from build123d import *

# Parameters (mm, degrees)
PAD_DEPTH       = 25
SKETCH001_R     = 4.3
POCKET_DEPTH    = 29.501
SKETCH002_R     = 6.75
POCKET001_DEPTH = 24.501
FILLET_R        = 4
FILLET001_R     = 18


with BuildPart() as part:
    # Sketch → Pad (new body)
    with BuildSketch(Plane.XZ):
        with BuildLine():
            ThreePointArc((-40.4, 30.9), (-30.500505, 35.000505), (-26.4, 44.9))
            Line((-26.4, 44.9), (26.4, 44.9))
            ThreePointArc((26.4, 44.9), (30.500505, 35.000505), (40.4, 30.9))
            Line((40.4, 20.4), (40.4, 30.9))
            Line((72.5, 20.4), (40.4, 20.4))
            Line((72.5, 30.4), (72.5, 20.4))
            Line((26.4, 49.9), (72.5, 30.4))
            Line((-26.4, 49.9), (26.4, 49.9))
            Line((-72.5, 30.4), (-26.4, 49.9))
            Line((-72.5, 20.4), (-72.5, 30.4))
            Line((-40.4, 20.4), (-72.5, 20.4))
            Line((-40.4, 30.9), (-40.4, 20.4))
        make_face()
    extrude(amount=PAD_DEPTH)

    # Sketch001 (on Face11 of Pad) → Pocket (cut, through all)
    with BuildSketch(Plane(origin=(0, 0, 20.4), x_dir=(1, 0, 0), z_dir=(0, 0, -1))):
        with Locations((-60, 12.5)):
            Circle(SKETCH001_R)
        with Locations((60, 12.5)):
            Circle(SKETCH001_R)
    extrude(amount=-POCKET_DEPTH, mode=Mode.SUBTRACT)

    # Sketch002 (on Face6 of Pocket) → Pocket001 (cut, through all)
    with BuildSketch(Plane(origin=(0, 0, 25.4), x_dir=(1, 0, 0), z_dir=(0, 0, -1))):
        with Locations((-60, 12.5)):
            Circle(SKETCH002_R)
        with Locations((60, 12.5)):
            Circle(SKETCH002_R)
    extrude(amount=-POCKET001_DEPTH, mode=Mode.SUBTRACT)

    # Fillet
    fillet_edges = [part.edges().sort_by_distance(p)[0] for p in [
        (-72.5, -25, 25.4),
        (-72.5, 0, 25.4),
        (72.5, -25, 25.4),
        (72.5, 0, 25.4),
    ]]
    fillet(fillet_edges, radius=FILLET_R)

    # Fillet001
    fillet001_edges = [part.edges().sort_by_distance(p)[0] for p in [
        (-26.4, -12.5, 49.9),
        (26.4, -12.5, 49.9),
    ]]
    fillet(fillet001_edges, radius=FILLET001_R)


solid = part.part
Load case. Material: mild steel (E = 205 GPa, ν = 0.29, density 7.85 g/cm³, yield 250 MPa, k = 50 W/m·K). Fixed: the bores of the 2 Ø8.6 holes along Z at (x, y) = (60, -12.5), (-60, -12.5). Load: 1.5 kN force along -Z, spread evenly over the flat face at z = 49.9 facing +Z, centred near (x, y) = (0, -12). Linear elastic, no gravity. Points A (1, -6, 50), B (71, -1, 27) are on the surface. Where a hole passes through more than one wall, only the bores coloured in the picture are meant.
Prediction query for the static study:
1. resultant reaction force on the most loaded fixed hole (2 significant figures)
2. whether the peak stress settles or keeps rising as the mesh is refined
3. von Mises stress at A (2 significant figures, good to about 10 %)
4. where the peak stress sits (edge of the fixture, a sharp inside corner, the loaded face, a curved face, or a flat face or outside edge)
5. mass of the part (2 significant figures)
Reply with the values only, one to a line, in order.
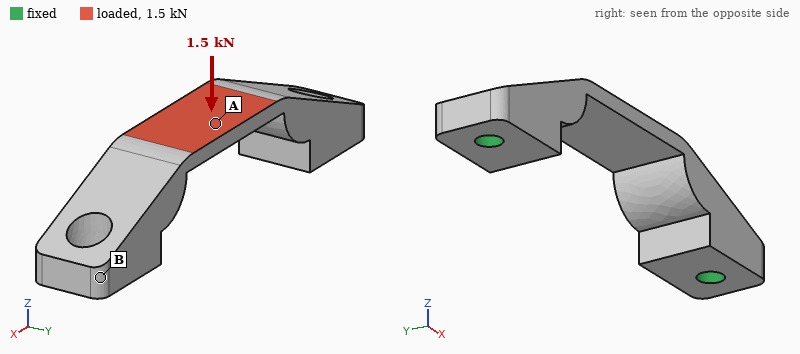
1.4 kN
keeps rising
55 MPa
a sharp inside corner
310 g
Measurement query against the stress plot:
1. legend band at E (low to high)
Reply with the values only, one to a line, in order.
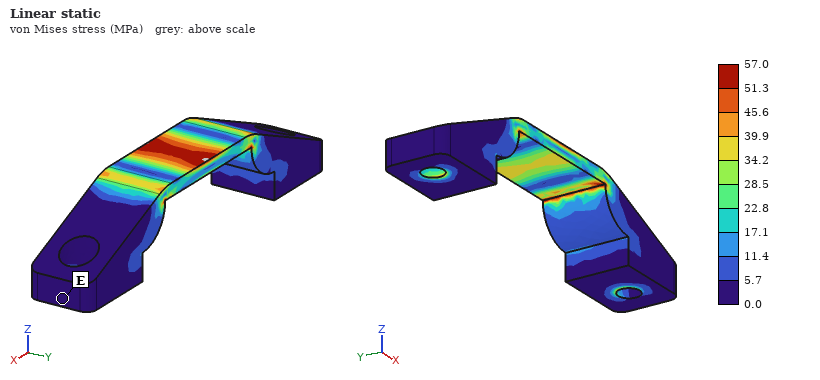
0.0 to 5.7 MPa
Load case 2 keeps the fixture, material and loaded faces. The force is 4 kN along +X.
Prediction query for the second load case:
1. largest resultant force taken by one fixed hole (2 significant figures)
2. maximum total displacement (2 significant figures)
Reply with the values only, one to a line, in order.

2.1 kN
30 µm
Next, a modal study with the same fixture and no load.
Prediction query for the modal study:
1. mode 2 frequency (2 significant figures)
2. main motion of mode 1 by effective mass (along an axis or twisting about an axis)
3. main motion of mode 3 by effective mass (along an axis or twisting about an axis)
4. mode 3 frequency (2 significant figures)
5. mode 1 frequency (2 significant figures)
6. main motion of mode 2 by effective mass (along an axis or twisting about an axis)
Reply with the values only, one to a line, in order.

4300 Hz
along Y
along Z
6400 Hz
4000 Hz
along X
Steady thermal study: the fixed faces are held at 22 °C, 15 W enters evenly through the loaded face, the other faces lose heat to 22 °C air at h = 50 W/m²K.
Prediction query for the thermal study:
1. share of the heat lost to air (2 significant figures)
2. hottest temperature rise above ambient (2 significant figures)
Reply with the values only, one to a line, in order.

37 %
33 K
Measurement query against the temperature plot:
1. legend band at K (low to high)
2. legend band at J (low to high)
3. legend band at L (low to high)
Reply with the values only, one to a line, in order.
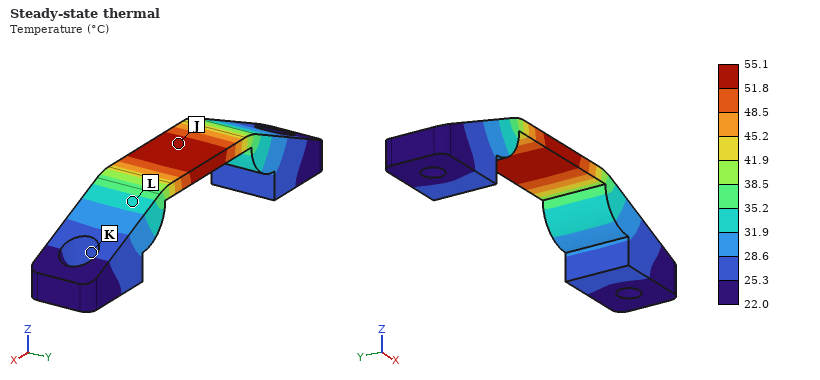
25.3 to 28.6 °C
51.8 to 55.1 °C
31.9 to 35.2 °C
